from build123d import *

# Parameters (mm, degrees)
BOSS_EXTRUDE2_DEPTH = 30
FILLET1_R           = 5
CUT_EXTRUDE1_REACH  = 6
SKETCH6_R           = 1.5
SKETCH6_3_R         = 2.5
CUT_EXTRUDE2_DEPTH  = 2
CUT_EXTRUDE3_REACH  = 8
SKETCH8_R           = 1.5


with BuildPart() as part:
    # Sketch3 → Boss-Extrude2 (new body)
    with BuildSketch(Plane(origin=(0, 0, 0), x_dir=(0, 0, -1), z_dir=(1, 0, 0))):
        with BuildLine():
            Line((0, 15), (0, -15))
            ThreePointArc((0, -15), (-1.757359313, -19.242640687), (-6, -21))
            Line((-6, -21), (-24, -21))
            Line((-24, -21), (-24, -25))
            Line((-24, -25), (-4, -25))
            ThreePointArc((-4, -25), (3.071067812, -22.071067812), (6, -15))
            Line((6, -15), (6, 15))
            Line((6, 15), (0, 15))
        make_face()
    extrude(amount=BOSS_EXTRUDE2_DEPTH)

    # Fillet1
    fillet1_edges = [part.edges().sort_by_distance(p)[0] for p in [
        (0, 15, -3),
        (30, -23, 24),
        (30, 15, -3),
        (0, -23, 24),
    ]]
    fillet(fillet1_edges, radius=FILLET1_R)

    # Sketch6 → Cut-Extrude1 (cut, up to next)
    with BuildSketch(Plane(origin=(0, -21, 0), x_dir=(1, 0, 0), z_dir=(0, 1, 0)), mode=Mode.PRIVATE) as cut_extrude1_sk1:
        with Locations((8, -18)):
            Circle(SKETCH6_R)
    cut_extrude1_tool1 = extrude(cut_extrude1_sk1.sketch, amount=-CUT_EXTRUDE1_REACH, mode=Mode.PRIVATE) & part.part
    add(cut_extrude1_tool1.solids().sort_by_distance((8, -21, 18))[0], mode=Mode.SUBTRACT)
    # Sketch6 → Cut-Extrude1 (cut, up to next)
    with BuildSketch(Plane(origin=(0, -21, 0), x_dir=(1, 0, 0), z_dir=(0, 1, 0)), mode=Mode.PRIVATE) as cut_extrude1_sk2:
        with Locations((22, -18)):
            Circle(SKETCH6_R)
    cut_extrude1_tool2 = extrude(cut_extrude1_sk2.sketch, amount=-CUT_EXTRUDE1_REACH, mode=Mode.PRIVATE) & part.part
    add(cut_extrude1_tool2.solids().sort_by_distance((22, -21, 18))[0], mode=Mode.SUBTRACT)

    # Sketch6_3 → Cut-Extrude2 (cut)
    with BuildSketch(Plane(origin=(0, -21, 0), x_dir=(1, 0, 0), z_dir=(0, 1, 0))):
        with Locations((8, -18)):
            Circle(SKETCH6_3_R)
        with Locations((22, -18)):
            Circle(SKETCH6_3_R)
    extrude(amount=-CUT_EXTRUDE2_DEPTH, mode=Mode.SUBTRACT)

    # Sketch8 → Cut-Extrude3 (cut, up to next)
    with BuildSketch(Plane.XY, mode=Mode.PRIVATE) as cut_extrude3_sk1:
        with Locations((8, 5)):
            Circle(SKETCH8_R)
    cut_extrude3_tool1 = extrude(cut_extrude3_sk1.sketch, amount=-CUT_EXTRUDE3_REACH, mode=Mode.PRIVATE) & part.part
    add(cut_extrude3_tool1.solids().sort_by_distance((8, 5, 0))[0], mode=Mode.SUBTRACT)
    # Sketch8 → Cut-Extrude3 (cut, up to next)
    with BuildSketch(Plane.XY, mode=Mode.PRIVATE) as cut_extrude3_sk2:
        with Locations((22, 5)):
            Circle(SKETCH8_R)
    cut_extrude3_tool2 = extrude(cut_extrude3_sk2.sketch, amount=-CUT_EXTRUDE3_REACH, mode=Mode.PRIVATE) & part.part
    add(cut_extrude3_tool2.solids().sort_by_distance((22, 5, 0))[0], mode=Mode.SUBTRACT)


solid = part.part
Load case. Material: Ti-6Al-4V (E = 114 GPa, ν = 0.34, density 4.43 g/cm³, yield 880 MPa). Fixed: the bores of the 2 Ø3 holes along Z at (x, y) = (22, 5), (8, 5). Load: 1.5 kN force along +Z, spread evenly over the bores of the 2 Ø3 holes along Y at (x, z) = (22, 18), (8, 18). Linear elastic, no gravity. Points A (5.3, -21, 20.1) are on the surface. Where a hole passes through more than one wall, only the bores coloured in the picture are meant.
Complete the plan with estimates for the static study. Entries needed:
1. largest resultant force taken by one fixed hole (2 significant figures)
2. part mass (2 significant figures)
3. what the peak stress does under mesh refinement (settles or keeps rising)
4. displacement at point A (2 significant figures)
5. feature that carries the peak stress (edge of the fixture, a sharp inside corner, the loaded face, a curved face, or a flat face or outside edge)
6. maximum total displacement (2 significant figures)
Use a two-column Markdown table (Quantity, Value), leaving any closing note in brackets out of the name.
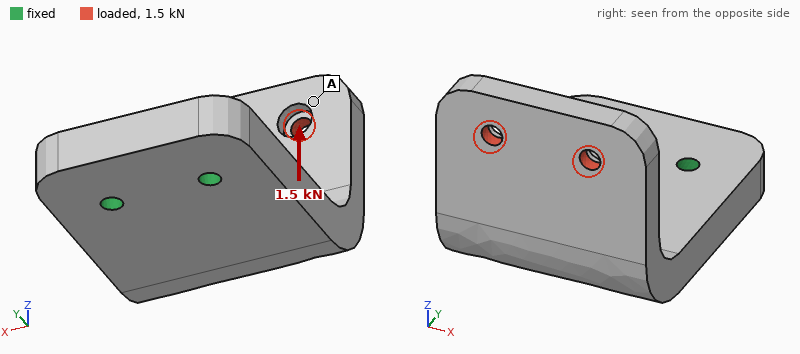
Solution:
| Quantity | Value |
|---|---|
| largest resultant force taken by one fixed hole | 750 N |
| part mass | 42 g |
| what the peak stress does under mesh refinement | keeps rising |
| displacement at point A | 0.32 mm |
| feature that carries the peak stress | edge of the fixture |
| maximum total displacement | 0.38 mm |
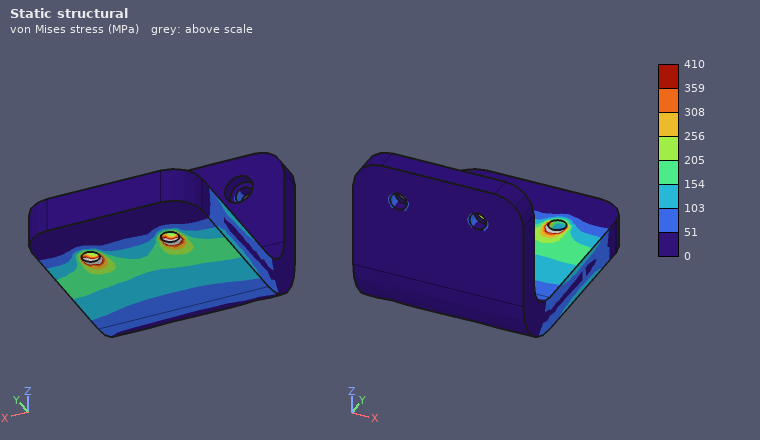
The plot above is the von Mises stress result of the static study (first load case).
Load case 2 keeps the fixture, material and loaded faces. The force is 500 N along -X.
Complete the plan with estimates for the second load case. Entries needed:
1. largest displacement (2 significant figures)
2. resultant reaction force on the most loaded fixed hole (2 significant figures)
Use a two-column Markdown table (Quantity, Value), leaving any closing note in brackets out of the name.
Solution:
| Quantity | Value |
|---|---|
| largest displacement | 83 µm |
| resultant reaction force on the most loaded fixed hole | 1.1 kN |
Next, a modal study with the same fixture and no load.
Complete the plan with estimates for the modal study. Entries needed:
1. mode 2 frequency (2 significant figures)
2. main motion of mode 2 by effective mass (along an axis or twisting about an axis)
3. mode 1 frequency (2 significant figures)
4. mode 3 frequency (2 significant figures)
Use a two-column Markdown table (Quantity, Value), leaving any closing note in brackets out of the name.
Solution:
| Quantity | Value |
|---|---|
| mode 2 frequency | 4500 Hz |
| main motion of mode 2 by effective mass | along X |
| mode 1 frequency | 2700 Hz |
| mode 3 frequency | 6600 Hz |
